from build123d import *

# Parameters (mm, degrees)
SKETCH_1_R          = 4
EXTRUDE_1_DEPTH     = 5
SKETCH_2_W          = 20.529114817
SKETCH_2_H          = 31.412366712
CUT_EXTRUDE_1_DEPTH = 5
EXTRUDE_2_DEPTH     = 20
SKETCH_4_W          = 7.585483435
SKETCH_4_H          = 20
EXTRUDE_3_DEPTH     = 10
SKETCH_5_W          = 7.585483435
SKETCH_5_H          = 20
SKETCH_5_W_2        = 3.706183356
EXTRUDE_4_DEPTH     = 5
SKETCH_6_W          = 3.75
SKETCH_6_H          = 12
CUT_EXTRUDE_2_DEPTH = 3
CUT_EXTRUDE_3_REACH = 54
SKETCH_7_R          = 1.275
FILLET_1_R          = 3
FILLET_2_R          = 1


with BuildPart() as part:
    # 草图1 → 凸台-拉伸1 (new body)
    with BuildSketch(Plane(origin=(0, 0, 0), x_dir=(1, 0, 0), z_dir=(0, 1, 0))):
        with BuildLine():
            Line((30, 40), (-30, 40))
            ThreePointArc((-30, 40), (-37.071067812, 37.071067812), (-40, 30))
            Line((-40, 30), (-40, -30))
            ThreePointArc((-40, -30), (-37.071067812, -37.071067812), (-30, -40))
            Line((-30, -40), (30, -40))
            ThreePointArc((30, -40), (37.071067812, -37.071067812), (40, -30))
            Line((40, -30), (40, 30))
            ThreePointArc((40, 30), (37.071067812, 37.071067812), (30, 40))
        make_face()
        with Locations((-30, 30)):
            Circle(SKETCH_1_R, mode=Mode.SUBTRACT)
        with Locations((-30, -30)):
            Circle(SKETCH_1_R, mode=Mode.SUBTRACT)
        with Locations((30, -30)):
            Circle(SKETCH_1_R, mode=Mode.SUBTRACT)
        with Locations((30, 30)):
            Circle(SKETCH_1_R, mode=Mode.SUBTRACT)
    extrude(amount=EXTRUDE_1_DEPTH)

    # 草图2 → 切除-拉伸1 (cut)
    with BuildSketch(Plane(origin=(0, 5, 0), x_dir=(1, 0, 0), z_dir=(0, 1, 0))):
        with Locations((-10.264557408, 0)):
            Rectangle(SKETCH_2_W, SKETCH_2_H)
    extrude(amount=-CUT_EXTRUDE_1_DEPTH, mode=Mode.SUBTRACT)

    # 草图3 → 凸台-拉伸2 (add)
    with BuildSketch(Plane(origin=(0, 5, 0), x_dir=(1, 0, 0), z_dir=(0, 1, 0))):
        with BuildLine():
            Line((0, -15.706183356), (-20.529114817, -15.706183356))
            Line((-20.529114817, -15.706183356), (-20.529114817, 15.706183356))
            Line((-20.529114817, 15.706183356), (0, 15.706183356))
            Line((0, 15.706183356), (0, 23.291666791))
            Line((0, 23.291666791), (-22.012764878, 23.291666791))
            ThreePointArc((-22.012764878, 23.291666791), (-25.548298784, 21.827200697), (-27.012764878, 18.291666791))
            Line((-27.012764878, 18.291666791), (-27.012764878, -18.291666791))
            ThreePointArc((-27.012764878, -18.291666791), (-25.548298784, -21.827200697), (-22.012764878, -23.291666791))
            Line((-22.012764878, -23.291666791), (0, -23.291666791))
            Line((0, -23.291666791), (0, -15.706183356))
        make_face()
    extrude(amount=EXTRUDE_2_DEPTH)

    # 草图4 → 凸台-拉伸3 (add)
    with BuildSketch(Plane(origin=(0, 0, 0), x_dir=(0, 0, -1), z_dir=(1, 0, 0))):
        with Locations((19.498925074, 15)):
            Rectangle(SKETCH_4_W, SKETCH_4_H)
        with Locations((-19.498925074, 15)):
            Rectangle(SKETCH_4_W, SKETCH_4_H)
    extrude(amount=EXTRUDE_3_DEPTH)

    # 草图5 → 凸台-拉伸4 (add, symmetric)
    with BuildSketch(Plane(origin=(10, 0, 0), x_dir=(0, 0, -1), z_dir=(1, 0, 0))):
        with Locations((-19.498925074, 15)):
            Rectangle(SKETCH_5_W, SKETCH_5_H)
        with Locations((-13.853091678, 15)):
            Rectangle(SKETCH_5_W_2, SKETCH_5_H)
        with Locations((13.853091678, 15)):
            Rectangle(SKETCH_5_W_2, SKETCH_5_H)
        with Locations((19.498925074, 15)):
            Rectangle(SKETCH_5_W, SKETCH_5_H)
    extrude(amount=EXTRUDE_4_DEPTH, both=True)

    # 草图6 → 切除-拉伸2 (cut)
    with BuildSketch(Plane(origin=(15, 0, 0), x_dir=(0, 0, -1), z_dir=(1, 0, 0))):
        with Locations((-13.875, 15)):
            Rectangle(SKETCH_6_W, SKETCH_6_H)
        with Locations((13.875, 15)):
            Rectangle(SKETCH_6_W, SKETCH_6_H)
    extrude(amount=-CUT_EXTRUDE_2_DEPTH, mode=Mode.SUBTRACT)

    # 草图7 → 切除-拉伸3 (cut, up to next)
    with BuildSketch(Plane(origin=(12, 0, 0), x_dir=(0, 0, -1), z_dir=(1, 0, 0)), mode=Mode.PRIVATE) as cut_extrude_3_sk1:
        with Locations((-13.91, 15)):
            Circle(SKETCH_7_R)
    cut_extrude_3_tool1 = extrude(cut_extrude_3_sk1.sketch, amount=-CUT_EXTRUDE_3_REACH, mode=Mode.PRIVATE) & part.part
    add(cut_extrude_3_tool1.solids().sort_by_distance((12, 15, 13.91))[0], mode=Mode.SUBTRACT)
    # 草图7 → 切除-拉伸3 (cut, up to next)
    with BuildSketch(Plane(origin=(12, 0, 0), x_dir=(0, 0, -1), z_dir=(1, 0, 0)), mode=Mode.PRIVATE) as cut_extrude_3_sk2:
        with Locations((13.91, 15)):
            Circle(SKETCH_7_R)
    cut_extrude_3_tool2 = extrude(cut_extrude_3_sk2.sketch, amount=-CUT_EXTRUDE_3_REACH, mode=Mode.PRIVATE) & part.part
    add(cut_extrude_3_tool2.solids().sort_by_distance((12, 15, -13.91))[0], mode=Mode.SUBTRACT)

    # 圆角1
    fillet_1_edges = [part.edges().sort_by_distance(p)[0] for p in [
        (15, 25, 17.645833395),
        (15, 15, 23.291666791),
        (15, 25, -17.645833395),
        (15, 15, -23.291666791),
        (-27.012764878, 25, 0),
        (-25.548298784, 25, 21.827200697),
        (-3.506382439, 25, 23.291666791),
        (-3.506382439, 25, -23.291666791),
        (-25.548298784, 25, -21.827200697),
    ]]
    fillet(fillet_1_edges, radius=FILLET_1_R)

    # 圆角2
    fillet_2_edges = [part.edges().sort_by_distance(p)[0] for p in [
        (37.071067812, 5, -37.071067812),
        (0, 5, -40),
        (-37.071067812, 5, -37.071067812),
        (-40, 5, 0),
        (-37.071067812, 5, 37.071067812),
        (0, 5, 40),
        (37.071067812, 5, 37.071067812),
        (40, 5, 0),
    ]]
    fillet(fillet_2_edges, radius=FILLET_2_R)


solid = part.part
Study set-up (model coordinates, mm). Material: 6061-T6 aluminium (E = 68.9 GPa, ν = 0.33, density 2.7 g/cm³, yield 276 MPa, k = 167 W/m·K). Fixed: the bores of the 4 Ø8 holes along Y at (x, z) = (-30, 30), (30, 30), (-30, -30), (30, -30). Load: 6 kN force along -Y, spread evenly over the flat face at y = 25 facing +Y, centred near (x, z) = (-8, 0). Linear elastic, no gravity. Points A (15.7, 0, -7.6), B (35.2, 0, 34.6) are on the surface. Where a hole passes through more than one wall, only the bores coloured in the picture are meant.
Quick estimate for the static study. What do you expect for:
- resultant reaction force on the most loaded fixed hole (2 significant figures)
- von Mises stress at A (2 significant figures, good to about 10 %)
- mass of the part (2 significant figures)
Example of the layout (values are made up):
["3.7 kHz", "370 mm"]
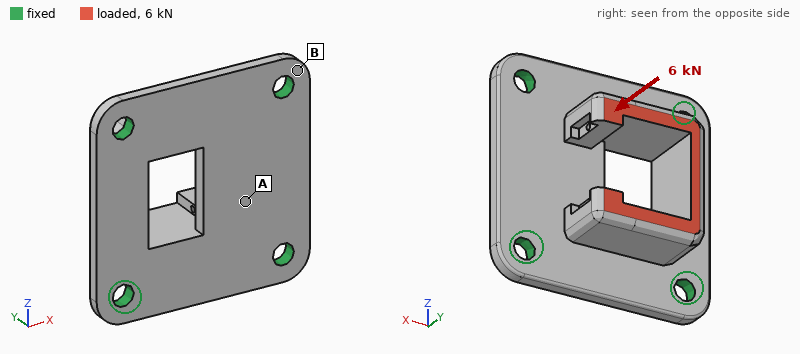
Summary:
["2.2 kN", "32 MPa", "120 g"]
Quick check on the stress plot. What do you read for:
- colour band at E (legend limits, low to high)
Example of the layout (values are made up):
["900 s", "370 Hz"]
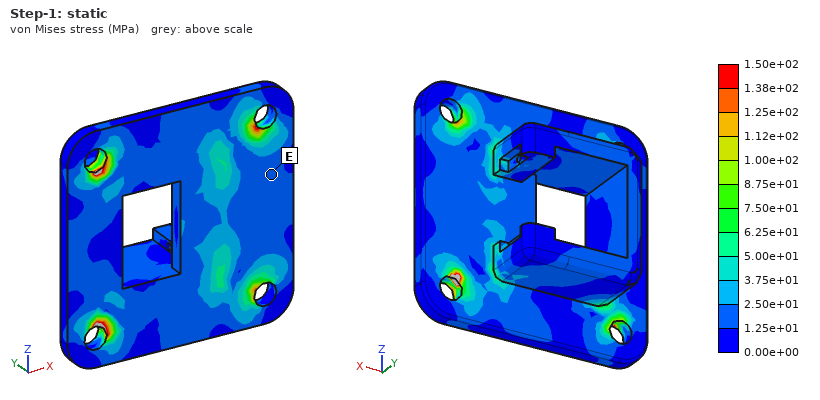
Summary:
["1.25e+01 to 2.50e+01 MPa"]
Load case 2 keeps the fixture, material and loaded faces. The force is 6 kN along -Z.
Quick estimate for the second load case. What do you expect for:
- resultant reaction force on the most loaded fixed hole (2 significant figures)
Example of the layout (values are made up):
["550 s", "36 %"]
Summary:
["2.9 kN"]
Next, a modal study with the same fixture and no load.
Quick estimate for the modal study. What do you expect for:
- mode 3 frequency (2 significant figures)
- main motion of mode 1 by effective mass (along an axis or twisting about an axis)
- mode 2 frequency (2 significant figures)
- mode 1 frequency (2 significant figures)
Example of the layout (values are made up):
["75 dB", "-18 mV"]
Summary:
["8600 Hz", "along Y", "8200 Hz", "5800 Hz"]
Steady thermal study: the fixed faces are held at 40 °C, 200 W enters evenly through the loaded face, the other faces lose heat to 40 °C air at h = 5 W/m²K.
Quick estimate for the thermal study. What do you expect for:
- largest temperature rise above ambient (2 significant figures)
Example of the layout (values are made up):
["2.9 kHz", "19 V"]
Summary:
["69 K"]
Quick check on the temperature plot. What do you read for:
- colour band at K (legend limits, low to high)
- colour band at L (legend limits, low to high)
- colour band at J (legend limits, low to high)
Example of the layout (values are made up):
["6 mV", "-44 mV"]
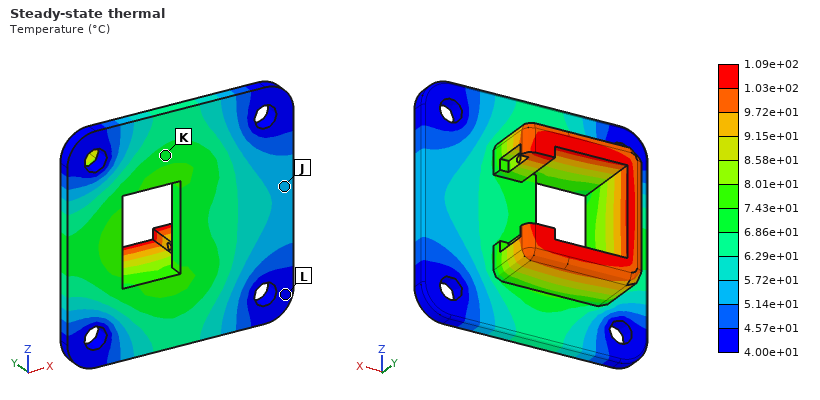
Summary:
["6.86e+01 to 7.43e+01 °C", "4.00e+01 to 4.57e+01 °C", "5.14e+01 to 5.72e+01 °C"]
